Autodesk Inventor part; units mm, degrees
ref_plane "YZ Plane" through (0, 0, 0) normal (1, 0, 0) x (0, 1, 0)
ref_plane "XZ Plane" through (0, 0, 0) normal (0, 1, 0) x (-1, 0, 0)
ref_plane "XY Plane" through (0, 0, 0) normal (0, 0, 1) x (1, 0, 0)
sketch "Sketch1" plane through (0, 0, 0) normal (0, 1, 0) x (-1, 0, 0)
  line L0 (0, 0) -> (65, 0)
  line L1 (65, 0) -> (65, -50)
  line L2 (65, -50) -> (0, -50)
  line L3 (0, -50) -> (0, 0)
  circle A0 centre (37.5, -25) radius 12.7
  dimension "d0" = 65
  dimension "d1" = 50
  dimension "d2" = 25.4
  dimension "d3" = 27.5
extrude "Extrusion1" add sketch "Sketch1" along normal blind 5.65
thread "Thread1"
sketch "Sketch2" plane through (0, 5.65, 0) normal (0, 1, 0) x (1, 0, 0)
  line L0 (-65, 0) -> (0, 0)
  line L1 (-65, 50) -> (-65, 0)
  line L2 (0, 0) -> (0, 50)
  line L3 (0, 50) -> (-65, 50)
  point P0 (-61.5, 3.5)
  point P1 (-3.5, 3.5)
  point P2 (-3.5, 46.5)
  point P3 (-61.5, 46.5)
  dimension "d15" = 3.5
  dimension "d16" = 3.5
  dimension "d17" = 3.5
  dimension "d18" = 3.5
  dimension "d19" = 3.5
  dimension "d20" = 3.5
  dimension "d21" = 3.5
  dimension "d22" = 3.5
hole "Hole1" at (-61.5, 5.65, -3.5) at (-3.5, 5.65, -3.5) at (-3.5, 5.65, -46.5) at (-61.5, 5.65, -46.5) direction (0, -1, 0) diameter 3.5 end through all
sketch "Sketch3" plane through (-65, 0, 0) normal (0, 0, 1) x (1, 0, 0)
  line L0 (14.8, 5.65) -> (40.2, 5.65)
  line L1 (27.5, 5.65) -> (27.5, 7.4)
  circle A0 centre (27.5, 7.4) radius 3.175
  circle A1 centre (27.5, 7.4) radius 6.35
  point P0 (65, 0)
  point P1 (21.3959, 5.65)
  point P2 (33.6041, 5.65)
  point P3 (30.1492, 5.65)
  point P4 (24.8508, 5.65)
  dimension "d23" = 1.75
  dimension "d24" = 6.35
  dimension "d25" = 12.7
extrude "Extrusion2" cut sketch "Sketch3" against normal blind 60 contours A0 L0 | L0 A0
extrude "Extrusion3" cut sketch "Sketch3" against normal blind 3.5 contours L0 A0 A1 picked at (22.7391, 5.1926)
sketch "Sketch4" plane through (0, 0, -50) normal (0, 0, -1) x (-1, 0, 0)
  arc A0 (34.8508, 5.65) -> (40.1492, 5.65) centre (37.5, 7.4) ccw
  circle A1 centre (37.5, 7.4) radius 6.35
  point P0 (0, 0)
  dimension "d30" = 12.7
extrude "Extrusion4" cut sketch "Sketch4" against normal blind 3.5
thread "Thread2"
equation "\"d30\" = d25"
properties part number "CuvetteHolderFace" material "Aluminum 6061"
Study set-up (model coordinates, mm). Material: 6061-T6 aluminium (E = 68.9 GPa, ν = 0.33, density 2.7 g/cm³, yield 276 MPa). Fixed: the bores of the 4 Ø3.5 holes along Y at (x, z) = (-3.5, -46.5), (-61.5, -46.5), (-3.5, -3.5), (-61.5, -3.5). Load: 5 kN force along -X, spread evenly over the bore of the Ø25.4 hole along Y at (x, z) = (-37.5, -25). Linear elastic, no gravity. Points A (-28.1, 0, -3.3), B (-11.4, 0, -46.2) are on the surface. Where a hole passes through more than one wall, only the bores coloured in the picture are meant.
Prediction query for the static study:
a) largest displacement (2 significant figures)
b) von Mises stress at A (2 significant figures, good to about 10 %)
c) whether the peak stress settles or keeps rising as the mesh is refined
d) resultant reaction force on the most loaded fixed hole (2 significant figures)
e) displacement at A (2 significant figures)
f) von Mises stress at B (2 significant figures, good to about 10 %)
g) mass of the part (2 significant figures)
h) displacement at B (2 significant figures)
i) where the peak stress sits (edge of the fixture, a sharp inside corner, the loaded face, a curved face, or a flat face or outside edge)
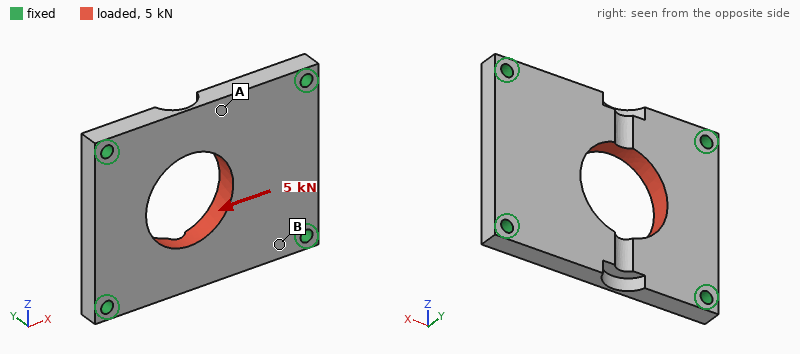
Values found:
12 µm
8.5 MPa
keeps rising
1.4 kN
4.9 µm
18 MPa
40 g
2.1 µm
edge of the fixture
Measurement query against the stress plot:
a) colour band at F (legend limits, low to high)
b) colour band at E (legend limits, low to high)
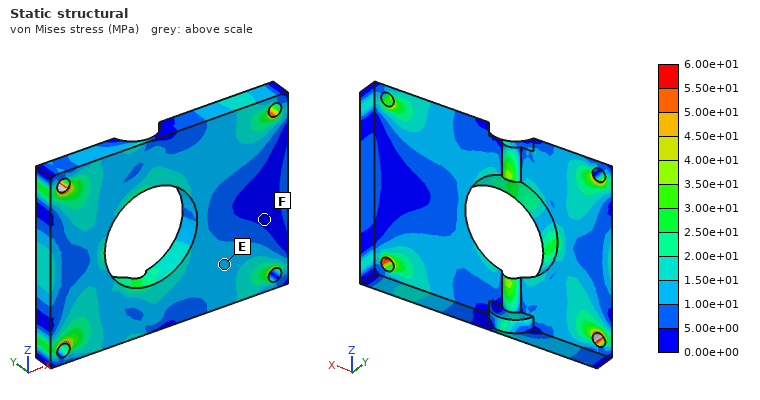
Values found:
0.00e+00 to 5.00e+00 MPa
1.00e+01 to 1.50e+01 MPa
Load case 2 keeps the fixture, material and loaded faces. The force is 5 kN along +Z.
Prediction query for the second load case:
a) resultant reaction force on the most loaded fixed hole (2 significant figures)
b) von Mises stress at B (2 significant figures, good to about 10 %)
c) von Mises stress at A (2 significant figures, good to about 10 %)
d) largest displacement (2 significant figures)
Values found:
1.5 kN
15 MPa
12 MPa
16 µm
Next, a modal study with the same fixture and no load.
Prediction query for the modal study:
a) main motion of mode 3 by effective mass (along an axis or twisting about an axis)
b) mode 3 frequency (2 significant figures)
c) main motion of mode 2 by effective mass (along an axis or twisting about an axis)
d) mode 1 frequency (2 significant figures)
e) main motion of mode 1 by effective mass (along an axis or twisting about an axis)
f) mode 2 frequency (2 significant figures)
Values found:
twisting about Z
13 kHz
twisting about X
6600 Hz
along Y
9600 Hz
